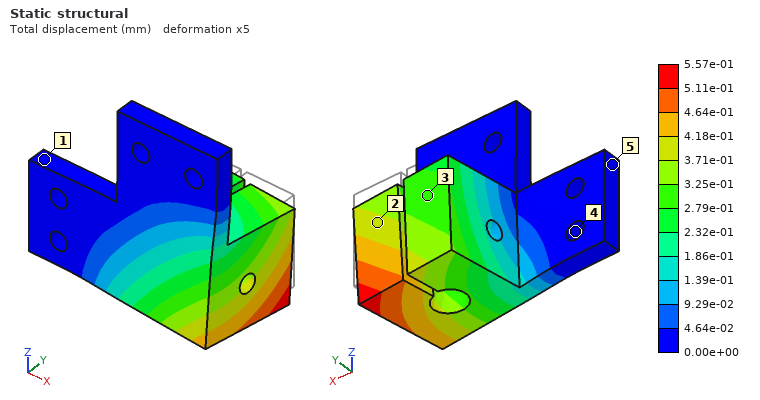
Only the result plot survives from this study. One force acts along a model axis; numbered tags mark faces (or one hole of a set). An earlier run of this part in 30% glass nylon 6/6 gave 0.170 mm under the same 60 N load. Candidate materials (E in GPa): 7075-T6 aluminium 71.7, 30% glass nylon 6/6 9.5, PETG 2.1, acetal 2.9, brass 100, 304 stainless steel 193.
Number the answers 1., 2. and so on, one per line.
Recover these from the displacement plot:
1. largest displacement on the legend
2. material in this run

1. 5.57e-01 mm
2. acetal
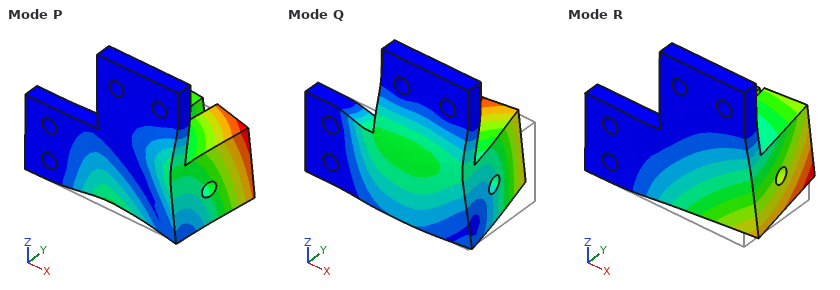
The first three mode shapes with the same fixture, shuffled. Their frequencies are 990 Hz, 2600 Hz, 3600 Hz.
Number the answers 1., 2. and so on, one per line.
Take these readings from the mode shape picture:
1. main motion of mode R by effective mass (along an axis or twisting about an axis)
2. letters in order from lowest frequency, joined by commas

1. along Y
2. R, P, Q
